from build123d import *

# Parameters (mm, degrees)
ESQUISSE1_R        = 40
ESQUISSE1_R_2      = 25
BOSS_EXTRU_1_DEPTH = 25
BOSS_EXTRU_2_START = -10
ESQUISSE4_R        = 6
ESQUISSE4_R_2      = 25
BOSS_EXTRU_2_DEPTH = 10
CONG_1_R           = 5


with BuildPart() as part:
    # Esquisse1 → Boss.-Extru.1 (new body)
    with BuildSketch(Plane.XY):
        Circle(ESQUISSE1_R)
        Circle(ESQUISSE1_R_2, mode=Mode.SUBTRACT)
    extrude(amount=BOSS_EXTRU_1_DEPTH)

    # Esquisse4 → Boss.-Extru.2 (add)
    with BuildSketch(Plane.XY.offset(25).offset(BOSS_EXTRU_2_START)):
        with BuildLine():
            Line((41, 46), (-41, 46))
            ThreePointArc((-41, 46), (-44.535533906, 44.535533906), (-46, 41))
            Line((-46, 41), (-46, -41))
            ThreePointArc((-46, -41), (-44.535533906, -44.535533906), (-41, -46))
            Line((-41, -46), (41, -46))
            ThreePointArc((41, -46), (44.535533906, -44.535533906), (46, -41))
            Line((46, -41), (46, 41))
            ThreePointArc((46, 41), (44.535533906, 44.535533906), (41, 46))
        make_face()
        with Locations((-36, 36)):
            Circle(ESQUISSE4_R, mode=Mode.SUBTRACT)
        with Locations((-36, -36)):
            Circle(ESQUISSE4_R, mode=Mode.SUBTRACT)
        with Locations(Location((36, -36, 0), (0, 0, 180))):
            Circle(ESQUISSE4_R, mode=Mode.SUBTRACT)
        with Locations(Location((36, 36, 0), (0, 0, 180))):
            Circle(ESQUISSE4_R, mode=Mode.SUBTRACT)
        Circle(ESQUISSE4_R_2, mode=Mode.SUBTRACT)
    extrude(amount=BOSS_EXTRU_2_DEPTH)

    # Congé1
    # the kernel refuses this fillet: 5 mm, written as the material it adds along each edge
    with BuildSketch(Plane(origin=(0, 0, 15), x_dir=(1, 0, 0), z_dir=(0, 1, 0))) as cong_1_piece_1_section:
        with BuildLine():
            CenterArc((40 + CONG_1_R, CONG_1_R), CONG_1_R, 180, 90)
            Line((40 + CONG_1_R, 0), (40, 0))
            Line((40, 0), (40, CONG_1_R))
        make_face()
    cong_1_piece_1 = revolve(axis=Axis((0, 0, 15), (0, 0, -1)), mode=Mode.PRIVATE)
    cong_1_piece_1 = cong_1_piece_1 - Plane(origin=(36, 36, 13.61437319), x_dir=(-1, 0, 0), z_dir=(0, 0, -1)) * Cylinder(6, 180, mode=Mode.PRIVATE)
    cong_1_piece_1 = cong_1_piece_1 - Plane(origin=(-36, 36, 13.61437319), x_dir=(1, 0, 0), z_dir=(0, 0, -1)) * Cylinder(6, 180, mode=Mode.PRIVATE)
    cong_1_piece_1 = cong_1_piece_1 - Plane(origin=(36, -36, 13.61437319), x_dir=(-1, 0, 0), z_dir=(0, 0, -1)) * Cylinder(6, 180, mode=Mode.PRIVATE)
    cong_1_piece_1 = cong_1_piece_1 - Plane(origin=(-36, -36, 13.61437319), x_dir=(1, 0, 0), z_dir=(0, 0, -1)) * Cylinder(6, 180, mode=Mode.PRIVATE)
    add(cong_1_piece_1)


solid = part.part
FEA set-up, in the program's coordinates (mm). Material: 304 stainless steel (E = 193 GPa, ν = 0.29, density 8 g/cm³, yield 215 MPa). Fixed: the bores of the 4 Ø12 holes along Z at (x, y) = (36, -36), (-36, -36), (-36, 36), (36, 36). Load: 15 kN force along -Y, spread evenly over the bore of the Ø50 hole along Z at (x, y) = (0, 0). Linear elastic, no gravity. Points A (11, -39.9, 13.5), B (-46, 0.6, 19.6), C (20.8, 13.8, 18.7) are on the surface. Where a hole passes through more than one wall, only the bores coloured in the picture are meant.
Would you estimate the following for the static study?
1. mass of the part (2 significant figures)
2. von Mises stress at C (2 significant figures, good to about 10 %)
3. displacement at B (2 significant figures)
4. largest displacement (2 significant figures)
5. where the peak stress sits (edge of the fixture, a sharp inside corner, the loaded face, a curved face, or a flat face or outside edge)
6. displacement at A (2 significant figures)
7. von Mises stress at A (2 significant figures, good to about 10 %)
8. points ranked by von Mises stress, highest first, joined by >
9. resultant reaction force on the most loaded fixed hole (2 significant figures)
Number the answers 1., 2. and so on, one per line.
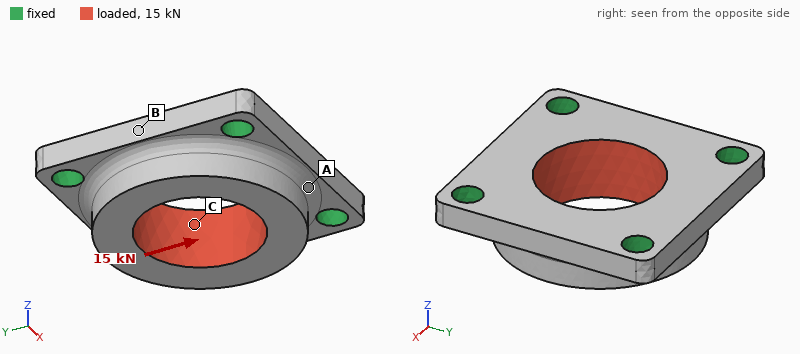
1. 860 g
2. 11 MPa
3. 1.2 µm
4. 4.1 µm
5. edge of the fixture
6. 2.7 µm
7. 6.7 MPa
8. C > A > B
9. 3.9 kN
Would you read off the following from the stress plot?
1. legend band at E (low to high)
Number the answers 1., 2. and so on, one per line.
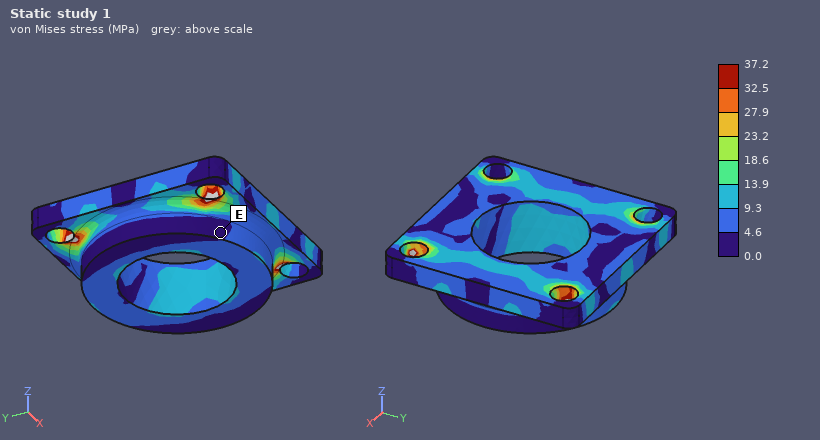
1. 0.0 to 4.6 MPa
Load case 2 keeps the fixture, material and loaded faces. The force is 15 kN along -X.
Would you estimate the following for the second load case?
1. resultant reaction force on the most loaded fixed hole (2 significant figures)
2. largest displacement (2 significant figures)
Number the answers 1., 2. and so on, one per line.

1. 3.9 kN
2. 4.1 µm
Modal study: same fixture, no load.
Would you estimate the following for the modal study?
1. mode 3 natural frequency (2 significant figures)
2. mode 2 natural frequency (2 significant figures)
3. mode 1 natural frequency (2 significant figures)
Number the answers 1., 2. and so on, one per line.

1. 13 kHz
2. 11 kHz
3. 11 kHz
